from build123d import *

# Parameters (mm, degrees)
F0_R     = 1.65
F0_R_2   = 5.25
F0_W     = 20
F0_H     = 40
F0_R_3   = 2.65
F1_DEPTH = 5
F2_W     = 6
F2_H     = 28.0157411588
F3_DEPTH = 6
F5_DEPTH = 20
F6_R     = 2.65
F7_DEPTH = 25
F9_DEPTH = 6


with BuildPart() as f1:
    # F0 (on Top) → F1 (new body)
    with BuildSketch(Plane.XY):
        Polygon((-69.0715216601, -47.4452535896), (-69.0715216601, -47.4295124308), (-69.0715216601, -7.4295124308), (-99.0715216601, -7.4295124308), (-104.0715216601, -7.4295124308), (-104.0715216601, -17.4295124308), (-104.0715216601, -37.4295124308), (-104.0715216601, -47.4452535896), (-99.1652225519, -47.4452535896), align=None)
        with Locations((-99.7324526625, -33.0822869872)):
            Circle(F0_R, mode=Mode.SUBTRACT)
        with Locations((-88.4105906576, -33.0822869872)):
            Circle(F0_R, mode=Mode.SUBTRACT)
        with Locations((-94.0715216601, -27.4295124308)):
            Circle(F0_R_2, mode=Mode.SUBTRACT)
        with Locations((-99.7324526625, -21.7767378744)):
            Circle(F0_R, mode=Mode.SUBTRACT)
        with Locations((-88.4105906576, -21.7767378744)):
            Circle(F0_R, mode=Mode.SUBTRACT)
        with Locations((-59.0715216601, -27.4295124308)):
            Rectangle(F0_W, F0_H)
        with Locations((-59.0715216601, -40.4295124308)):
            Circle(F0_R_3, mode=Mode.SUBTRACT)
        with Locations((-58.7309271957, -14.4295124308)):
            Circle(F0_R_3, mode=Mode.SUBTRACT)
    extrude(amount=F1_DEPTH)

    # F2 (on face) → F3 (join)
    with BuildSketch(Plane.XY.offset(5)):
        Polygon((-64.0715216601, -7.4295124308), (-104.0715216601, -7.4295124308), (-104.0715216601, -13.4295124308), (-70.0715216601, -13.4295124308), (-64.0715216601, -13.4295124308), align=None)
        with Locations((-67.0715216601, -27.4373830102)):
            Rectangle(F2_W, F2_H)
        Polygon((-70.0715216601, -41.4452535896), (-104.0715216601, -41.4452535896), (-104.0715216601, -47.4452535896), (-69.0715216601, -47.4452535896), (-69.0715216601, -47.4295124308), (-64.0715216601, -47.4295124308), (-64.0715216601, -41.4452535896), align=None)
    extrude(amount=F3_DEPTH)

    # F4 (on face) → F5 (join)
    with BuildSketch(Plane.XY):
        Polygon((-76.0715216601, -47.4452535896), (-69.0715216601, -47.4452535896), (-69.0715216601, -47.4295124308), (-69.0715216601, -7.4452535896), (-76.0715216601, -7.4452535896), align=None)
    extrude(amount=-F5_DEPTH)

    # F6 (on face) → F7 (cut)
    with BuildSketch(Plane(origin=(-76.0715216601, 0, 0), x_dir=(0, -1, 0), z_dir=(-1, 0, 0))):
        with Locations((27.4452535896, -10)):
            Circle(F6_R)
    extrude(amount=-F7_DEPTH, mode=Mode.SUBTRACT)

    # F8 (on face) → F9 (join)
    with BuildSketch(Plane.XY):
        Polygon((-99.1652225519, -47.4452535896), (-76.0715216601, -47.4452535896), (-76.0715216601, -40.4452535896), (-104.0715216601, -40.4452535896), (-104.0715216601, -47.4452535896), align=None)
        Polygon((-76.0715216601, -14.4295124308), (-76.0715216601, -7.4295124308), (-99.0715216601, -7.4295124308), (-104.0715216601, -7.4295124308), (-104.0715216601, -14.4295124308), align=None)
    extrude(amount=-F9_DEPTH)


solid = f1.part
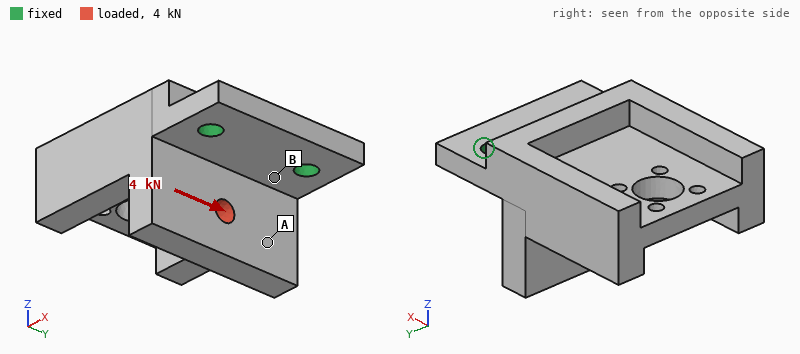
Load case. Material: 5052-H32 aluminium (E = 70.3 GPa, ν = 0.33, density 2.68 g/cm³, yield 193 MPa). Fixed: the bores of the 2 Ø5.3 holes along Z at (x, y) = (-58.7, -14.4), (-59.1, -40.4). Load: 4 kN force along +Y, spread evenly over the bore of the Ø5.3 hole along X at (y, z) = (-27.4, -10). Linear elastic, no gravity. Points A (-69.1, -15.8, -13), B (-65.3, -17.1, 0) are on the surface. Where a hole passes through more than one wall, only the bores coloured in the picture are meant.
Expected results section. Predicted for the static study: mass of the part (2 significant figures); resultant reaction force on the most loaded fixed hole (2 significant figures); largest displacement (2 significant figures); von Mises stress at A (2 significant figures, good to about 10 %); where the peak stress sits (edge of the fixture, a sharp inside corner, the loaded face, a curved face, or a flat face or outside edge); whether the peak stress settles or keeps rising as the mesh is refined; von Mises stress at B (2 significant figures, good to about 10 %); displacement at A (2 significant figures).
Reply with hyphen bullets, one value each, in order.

- 59 g
- 3.2 kN
- 92 µm
- 19 MPa
- edge of the fixture
- keeps rising
- 81 MPa
- 56 µm
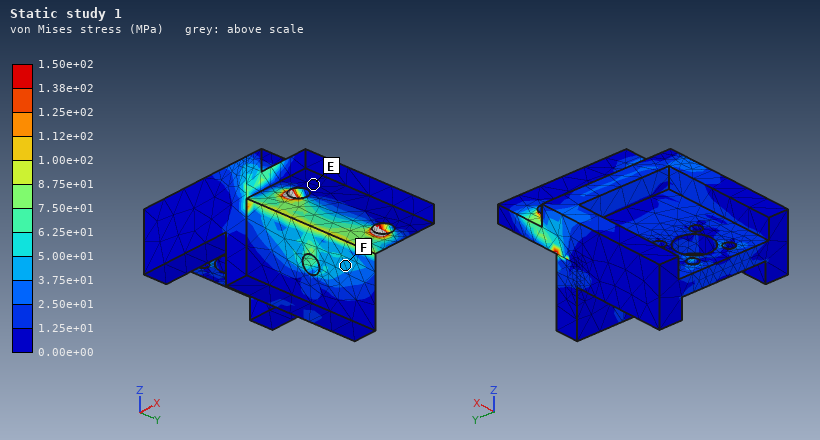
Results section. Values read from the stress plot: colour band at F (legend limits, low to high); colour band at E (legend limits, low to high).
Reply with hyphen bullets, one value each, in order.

- 3.75e+01 to 5.00e+01 MPa
- 0.00e+00 to 1.25e+01 MPa
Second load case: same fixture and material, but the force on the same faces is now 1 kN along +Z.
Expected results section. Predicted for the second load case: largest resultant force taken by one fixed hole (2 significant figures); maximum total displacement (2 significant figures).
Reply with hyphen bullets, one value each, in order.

- 510 N
- 0.10 mm
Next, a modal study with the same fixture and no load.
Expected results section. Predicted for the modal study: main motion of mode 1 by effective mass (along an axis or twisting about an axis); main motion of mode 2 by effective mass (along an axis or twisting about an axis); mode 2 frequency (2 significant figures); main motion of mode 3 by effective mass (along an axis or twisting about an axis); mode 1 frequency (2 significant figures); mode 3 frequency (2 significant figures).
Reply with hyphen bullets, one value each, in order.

- along Z
- twisting about X
- 4900 Hz
- along Y
- 1900 Hz
- 8200 Hz
